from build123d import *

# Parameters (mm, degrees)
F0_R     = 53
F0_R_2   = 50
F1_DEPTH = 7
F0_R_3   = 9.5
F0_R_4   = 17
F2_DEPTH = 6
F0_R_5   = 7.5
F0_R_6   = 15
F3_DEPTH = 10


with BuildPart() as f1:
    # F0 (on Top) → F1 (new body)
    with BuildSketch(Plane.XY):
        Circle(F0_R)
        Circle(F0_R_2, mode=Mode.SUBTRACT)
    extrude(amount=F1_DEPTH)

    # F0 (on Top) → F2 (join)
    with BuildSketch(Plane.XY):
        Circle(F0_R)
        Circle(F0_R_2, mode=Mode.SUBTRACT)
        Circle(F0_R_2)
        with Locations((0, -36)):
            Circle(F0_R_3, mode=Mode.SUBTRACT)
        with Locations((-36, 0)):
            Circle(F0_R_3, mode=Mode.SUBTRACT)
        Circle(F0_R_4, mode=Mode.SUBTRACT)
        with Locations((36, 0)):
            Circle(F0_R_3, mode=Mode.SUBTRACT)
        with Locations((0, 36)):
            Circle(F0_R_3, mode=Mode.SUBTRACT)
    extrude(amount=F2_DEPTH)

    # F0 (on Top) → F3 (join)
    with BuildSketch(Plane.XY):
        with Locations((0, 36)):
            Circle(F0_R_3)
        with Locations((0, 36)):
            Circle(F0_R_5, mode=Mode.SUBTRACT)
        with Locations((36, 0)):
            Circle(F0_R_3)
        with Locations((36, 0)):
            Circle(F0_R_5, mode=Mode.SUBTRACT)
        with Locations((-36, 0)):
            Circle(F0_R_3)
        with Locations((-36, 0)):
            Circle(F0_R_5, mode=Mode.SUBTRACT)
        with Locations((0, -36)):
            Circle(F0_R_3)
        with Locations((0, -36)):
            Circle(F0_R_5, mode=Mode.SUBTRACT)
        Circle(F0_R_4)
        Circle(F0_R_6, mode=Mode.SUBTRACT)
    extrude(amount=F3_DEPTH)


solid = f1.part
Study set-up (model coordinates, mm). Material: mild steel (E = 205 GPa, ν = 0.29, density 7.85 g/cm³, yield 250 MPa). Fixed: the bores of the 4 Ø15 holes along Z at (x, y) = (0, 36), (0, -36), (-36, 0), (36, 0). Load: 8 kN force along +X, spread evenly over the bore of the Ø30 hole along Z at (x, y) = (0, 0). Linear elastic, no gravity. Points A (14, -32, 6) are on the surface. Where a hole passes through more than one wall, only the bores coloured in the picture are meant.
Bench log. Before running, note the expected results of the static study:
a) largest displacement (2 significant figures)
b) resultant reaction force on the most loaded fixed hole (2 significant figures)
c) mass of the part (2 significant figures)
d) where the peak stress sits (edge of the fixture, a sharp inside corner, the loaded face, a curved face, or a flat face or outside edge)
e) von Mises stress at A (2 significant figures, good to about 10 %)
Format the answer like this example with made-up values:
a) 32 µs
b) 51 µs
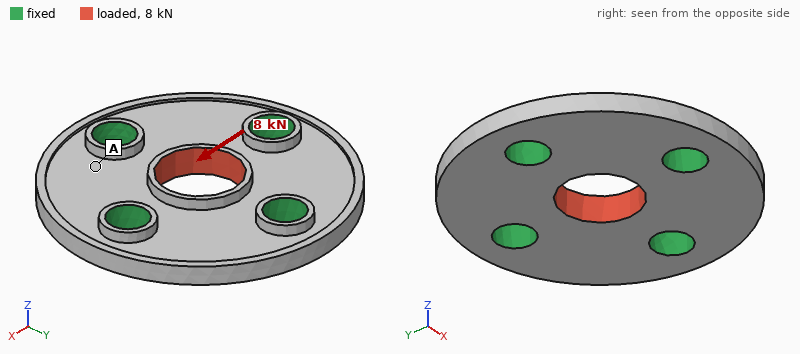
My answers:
a) 4.3 µm
b) 2.5 kN
c) 380 g
d) the loaded face
e) 5.6 MPa
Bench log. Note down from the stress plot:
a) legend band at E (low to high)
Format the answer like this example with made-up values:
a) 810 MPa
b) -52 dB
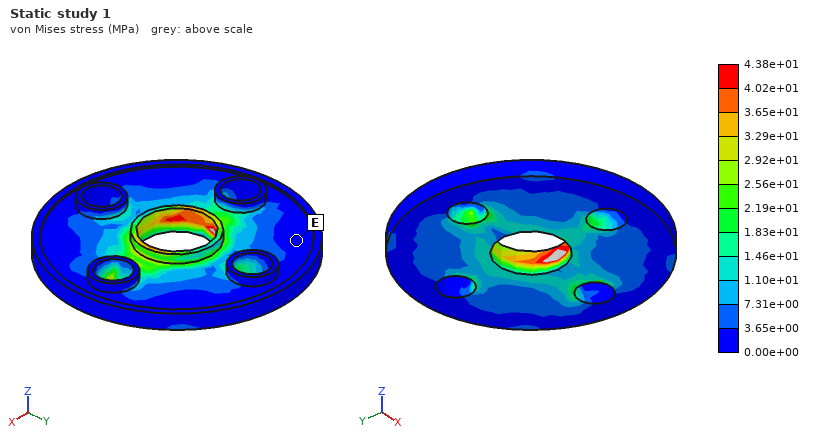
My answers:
a) 0.00e+00 to 3.65e+00 MPa
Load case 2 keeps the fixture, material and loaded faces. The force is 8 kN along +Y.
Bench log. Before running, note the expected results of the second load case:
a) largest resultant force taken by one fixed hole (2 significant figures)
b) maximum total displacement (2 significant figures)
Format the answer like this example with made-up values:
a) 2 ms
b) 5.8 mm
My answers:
a) 2.5 kN
b) 4.4 µm
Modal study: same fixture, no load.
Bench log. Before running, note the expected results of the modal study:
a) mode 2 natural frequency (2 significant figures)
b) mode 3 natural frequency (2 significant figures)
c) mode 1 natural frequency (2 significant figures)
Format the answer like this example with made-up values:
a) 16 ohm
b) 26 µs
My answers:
a) 9400 Hz
b) 9400 Hz
c) 9300 Hz
